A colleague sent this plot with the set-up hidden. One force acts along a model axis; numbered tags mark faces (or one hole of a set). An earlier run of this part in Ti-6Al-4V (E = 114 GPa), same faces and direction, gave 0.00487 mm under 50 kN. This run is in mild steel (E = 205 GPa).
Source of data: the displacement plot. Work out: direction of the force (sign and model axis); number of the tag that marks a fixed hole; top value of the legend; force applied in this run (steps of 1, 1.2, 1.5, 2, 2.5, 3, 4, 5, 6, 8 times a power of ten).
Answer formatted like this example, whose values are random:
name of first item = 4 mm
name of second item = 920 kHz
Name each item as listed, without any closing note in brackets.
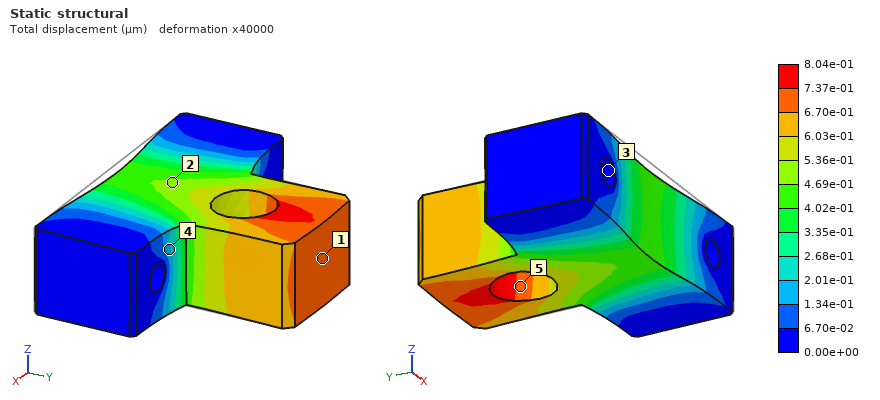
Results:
direction of the force = +Y
number of the tag that marks a fixed hole = 3
top value of the legend = 8.04e-01 µm
force applied in this run = 15 kN
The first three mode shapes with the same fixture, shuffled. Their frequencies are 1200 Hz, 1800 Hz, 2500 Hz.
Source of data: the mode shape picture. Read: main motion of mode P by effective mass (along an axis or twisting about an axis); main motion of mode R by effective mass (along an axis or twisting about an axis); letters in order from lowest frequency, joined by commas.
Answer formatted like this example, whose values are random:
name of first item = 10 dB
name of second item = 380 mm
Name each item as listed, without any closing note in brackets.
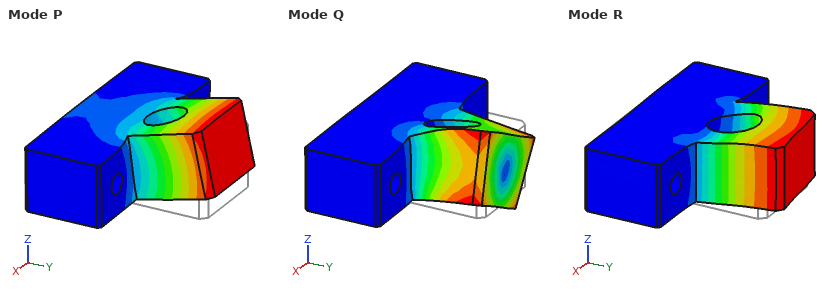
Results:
main motion of mode P by effective mass = along Z
main motion of mode R by effective mass = along X
letters in order from lowest frequency, joined by commas = P, R, Q
